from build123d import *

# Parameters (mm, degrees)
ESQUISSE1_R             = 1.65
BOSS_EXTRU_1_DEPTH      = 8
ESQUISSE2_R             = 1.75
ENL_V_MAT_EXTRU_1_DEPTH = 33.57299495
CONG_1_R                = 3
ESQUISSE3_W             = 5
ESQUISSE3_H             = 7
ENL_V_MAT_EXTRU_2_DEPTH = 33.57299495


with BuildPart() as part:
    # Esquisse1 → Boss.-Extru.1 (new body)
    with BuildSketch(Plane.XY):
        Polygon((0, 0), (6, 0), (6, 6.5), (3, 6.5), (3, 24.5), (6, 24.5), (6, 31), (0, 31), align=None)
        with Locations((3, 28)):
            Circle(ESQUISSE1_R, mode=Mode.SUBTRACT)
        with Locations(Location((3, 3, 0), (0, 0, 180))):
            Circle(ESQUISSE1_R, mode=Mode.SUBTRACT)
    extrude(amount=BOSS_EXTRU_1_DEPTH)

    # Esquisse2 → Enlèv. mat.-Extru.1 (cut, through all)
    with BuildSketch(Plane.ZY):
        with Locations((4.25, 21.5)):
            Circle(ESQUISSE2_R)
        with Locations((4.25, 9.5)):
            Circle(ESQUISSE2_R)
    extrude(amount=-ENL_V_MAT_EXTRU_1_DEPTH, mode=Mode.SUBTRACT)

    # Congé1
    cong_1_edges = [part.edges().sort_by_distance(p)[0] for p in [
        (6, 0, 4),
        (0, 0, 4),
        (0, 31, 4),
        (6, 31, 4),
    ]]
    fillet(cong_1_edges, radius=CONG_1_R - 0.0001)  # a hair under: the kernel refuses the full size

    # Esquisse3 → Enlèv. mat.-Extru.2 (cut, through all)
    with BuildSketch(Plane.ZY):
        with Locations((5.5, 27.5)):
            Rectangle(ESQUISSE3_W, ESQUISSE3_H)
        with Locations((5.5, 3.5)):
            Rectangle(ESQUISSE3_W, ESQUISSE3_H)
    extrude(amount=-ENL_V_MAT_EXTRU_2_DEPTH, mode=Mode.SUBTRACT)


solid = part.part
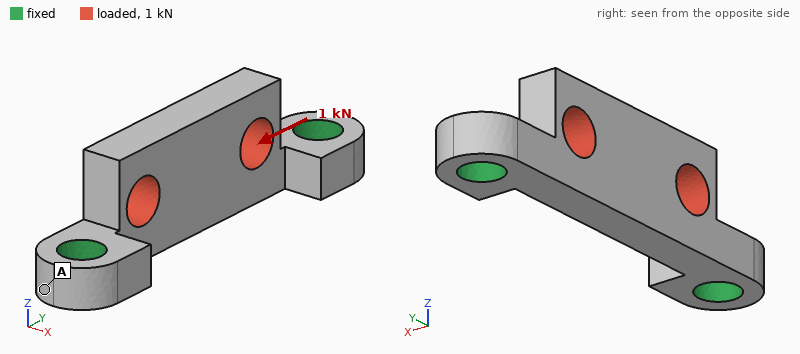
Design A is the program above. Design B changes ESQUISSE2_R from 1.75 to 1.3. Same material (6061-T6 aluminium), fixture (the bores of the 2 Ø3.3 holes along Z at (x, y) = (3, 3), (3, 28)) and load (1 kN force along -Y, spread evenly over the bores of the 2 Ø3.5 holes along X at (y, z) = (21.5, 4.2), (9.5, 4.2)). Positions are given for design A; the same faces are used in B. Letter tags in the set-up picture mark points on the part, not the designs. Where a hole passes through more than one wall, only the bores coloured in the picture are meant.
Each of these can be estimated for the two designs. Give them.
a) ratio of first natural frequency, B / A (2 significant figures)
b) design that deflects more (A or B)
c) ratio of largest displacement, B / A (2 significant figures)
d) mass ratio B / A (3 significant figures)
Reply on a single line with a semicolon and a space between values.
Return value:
1.0; A; 0.69; 1.05
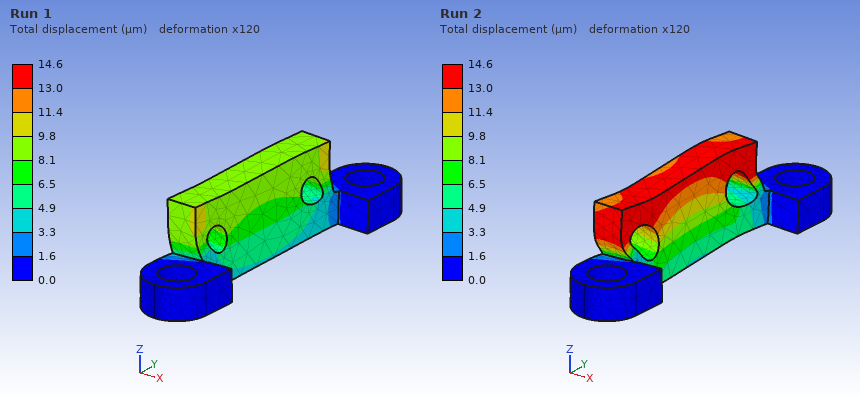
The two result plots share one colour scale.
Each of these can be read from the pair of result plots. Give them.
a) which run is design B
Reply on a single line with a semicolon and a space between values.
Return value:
Run 1
